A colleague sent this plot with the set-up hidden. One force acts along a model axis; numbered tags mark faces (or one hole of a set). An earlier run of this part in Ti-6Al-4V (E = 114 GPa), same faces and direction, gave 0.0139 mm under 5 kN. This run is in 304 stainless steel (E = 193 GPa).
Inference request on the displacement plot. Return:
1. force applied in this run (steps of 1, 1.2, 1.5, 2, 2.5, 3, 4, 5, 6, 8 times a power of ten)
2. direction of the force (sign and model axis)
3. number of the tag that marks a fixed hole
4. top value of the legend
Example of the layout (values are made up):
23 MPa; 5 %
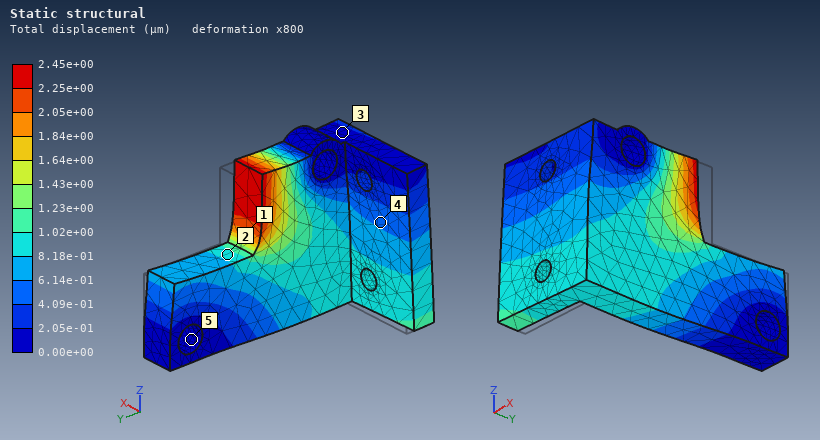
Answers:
1.5 kN; -Y; 5; 2.45e+00 µm
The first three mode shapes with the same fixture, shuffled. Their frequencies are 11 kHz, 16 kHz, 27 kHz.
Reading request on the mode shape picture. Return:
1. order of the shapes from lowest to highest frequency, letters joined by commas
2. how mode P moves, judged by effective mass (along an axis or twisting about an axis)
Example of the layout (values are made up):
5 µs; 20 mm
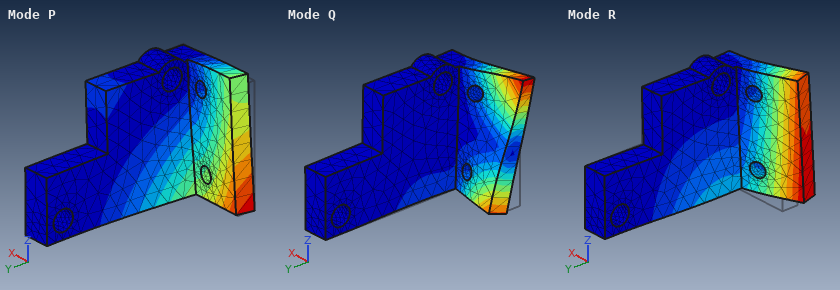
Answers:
P, R, Q; along X
